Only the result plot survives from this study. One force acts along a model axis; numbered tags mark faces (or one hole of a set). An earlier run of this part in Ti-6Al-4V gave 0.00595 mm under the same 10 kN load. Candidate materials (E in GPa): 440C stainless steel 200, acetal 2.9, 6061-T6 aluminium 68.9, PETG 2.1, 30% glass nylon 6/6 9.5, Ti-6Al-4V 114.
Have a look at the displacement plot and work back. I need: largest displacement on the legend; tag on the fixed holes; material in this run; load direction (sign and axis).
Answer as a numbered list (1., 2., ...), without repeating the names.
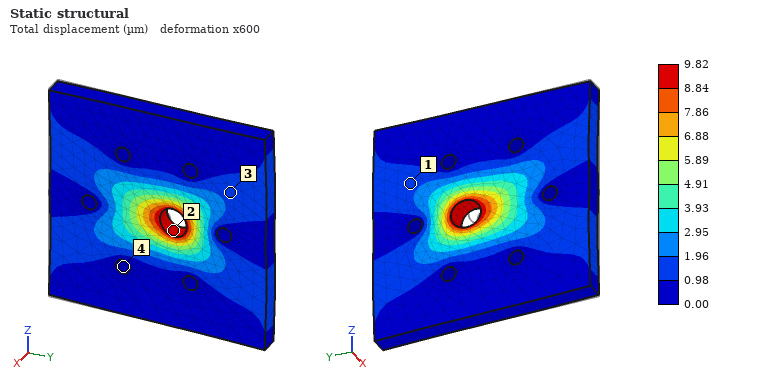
1. 9.82 µm
2. 4
3. 6061-T6 aluminium
4. +Y
